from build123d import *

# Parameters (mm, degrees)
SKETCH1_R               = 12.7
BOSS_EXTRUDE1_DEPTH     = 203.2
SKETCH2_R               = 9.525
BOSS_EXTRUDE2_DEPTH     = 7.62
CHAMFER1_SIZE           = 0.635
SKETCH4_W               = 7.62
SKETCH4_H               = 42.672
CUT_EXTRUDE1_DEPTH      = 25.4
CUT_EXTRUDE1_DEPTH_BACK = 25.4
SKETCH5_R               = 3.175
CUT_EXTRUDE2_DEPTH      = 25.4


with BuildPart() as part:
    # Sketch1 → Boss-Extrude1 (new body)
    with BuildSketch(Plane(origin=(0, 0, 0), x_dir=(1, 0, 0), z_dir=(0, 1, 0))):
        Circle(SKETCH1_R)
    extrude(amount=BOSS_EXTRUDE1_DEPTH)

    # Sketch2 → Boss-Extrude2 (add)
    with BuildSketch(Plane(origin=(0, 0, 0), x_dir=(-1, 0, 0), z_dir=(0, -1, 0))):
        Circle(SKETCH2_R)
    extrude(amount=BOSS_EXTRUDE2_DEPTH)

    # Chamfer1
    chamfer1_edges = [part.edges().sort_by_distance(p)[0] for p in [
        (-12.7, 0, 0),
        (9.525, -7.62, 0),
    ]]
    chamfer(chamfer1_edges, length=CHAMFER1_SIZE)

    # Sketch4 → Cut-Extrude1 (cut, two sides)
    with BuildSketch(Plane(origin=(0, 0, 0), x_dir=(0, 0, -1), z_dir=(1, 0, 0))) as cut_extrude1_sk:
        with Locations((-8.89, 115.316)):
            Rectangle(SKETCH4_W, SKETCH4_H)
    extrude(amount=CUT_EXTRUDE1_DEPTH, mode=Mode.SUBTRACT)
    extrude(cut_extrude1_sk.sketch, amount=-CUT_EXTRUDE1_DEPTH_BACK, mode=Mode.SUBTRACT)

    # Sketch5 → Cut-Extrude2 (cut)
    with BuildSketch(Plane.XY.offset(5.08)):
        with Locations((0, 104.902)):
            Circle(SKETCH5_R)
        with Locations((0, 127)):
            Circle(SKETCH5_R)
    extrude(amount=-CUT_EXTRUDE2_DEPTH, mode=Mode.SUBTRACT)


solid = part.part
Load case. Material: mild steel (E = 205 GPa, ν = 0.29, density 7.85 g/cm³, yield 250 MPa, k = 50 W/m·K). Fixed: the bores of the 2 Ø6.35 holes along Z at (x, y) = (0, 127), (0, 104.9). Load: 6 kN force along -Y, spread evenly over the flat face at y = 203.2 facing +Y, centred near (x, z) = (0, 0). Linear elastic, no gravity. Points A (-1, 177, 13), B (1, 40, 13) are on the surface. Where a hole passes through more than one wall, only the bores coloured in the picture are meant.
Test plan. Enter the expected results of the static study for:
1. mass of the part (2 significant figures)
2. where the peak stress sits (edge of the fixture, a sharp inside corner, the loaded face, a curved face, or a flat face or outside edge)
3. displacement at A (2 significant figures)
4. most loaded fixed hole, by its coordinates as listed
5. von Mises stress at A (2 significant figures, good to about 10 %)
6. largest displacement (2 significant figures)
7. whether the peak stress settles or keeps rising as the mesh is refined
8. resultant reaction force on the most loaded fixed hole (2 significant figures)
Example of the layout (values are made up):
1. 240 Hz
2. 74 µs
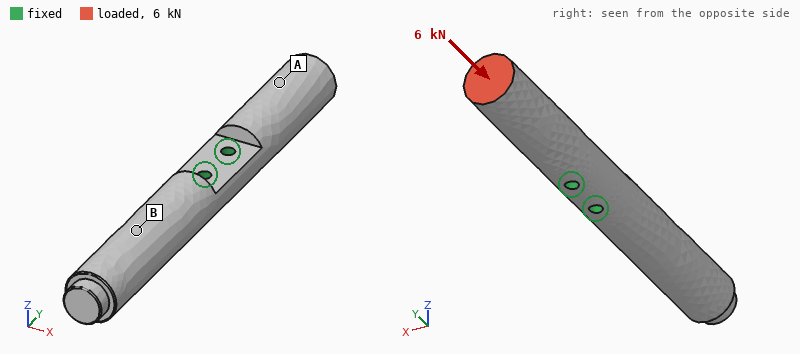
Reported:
1. 770 g
2. edge of the fixture
3. 8.8 µm
4. (0, 127)
5. 12 MPa
6. 13 µm
7. keeps rising
8. 5.2 kN
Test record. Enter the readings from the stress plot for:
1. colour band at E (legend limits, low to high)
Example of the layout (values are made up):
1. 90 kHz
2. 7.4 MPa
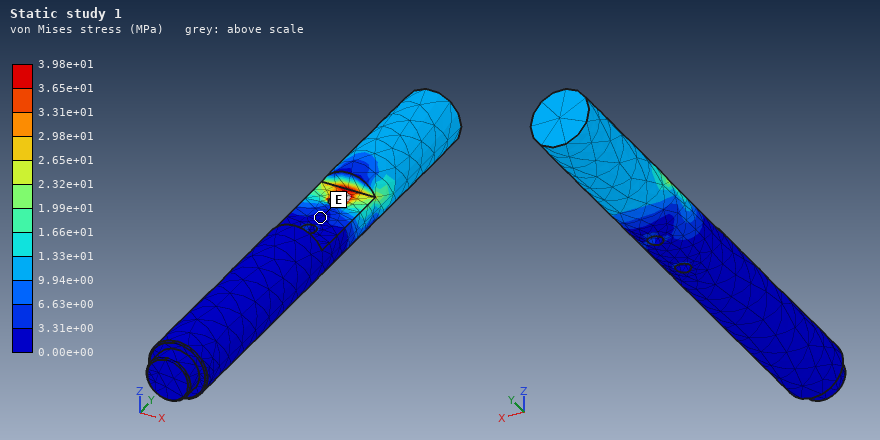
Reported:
1. 0.00e+00 to 3.31e+00 MPa
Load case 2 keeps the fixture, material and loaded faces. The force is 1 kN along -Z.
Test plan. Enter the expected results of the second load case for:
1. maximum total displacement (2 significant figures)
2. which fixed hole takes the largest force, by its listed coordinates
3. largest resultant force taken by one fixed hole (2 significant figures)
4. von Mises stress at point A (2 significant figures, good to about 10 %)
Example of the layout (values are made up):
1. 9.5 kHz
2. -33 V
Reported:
1. 62 µm
2. (0, 127)
3. 1.5 kN
4. 16 MPa
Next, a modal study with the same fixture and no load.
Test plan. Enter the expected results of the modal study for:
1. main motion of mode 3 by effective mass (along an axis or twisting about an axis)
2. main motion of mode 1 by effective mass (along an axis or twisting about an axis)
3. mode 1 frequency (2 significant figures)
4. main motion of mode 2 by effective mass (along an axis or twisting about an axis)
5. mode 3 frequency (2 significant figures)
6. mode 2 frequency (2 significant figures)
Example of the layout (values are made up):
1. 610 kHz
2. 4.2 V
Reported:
1. along Z
2. along Z
3. 1200 Hz
4. along X
5. 2200 Hz
6. 1200 Hz
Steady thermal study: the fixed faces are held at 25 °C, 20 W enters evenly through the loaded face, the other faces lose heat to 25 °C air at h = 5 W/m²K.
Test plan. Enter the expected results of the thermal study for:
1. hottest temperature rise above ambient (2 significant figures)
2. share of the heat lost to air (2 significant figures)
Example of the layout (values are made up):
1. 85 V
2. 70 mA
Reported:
1. 61 K
2. 4.9 %
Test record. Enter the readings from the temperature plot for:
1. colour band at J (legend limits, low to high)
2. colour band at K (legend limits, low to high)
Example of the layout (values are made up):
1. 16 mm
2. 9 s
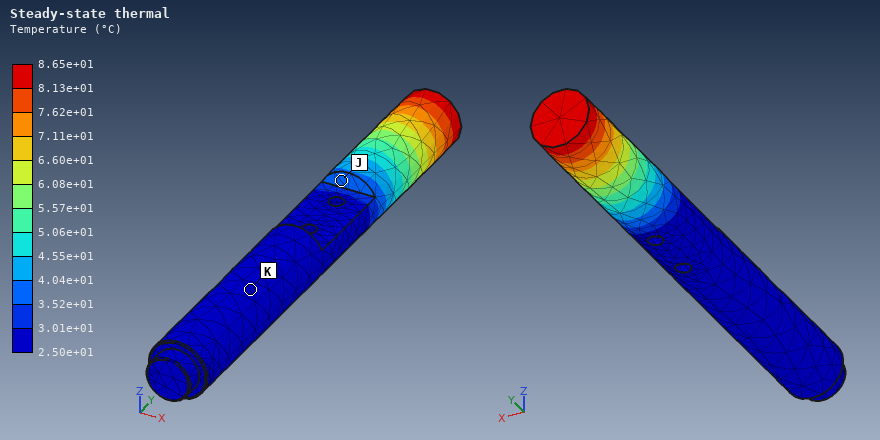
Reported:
1. 3.52e+01 to 4.04e+01 °C
2. 2.50e+01 to 3.01e+01 °C
